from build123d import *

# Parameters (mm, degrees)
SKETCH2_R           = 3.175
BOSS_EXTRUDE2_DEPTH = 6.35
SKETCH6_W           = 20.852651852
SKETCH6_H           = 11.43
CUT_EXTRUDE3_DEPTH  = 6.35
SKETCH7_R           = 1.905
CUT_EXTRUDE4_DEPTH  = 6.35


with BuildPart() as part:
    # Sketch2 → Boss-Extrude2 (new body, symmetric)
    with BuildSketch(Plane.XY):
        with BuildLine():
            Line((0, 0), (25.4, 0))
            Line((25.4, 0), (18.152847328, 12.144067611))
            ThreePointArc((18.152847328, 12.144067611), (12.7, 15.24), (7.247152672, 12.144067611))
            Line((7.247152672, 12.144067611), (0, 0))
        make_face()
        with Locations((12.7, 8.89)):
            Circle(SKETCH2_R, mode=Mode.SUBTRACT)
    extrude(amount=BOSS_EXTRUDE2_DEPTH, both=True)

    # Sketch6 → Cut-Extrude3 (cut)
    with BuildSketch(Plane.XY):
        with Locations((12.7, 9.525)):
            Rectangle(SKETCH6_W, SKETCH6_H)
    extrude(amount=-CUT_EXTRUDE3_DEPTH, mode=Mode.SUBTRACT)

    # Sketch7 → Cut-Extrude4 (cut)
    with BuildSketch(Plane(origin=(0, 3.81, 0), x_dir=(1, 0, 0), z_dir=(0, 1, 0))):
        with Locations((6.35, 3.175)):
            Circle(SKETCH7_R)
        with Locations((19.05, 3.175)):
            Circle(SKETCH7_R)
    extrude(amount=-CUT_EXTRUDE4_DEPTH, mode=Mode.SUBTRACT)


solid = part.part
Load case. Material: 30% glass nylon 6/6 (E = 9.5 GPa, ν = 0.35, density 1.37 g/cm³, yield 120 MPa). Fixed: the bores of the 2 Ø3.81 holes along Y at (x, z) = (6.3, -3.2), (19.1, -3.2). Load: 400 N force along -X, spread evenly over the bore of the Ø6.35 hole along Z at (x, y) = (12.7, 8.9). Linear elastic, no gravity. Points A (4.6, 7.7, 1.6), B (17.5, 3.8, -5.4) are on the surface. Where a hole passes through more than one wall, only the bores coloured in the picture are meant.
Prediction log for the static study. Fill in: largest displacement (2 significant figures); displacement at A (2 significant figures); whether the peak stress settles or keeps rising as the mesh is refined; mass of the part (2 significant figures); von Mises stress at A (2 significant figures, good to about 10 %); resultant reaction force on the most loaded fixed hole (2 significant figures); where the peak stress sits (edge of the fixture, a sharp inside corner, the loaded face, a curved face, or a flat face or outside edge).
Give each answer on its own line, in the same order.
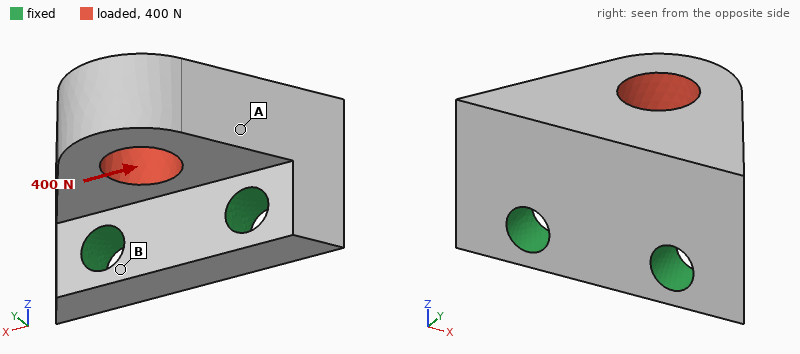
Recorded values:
47 µm
27 µm
keeps rising
2.5 g
12 MPa
300 N
edge of the fixture
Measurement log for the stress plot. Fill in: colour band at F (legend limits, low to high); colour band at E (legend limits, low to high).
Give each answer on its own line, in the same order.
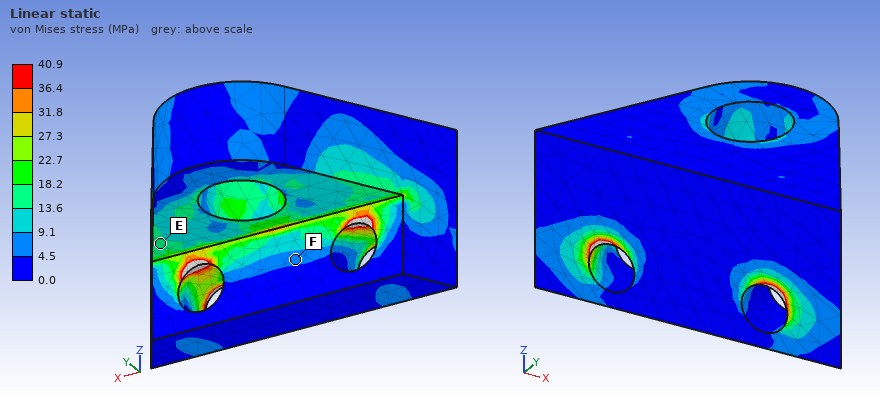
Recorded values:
4.5 to 9.1 MPa
13.6 to 18.2 MPa
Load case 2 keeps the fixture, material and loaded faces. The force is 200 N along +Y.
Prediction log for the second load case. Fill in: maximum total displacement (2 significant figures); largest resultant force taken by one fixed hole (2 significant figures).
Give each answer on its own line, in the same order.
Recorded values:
52 µm
100 N
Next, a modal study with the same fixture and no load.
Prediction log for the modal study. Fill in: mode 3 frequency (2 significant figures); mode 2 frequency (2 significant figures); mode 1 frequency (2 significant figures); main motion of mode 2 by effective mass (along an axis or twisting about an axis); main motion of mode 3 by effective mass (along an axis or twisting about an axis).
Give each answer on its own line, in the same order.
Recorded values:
23 kHz
15 kHz
7700 Hz
along X
along Y
